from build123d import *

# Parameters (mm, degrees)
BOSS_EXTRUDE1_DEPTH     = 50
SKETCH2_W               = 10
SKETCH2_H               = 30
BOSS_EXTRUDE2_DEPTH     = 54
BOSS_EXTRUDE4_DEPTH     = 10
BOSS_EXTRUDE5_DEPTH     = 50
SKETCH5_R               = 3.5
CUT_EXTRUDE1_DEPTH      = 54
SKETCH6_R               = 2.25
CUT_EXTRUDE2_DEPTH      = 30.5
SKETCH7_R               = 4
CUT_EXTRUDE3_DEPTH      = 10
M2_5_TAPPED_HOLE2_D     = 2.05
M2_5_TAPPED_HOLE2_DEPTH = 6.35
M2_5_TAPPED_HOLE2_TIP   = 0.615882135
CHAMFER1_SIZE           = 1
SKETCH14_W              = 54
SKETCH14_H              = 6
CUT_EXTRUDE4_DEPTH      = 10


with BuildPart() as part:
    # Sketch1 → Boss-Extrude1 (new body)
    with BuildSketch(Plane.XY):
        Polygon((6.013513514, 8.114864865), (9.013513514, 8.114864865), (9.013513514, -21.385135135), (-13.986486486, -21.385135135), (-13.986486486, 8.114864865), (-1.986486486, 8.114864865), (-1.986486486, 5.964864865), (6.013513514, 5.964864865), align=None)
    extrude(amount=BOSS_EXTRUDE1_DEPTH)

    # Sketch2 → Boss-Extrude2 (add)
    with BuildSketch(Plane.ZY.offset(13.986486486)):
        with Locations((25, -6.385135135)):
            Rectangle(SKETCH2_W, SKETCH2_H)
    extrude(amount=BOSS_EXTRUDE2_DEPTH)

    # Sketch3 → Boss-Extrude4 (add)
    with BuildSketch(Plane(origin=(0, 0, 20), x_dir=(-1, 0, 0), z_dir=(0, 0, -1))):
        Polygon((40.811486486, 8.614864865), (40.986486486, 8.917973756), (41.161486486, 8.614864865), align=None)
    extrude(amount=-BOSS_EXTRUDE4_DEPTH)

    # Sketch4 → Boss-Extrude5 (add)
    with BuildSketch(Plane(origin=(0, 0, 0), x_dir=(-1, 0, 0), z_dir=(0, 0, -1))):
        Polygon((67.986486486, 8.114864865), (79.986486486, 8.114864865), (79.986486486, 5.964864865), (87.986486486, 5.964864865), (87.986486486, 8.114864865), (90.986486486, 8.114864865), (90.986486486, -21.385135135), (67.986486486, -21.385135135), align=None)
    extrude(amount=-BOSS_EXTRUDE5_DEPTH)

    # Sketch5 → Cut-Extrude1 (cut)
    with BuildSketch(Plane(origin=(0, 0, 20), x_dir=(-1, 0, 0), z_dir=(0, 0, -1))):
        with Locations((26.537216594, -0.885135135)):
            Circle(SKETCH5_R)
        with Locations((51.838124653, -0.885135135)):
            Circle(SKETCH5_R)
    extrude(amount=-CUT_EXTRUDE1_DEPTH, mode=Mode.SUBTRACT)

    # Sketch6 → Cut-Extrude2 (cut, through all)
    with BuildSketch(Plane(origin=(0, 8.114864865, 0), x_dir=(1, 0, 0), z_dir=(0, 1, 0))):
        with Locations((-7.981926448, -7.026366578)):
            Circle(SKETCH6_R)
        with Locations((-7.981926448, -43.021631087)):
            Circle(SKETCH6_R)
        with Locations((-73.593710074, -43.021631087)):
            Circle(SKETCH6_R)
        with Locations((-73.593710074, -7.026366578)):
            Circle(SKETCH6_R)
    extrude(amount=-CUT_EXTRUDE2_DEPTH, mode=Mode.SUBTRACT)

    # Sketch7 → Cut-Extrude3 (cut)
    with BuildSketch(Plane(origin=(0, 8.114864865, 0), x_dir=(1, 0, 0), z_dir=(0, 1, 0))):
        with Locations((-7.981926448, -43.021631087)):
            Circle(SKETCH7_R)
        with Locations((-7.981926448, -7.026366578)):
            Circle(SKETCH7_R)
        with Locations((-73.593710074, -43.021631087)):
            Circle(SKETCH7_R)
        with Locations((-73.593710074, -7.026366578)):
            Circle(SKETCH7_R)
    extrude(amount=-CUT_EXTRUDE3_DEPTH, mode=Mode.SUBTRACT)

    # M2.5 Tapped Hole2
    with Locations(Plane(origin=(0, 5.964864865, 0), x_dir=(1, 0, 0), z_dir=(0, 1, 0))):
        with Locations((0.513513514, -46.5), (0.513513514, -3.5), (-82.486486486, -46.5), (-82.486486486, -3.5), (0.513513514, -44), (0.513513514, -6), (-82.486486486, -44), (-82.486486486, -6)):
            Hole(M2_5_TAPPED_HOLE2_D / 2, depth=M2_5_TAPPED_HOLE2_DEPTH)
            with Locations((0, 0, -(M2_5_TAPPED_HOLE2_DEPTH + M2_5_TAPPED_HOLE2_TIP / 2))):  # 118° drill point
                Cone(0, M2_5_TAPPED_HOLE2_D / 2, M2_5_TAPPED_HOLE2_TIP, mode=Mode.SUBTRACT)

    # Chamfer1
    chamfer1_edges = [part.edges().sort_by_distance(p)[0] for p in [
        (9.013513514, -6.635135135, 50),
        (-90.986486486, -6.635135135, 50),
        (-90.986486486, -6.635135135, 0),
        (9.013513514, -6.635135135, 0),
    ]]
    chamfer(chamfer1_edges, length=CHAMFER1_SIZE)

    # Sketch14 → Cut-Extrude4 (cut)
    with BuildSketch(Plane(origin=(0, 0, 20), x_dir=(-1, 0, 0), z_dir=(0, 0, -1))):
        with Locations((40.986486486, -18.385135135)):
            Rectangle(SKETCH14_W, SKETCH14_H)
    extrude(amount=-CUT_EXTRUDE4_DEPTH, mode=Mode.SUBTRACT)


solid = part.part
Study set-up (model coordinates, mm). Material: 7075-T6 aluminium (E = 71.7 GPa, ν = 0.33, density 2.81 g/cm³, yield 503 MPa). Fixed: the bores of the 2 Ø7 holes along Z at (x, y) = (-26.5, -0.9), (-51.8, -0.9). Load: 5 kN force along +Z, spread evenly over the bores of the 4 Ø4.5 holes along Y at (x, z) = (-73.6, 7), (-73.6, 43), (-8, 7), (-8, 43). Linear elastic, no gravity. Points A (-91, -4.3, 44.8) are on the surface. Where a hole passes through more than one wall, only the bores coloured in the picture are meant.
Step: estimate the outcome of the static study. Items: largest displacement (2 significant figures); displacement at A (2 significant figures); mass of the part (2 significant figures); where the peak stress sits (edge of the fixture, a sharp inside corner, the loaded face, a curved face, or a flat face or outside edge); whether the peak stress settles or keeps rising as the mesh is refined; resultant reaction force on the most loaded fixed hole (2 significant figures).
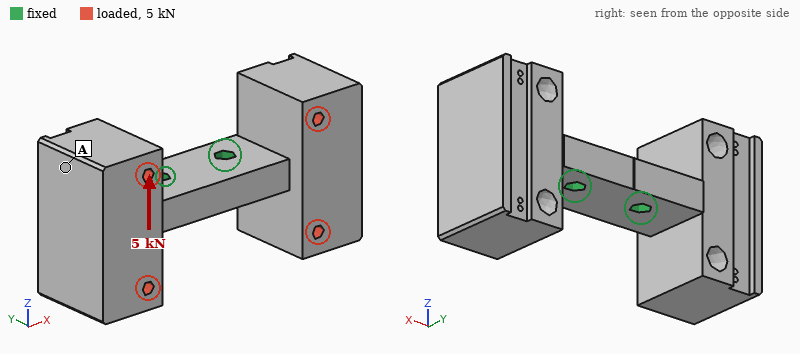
0.20 mm
0.16 mm
210 g
edge of the fixture
keeps rising
2.6 kN
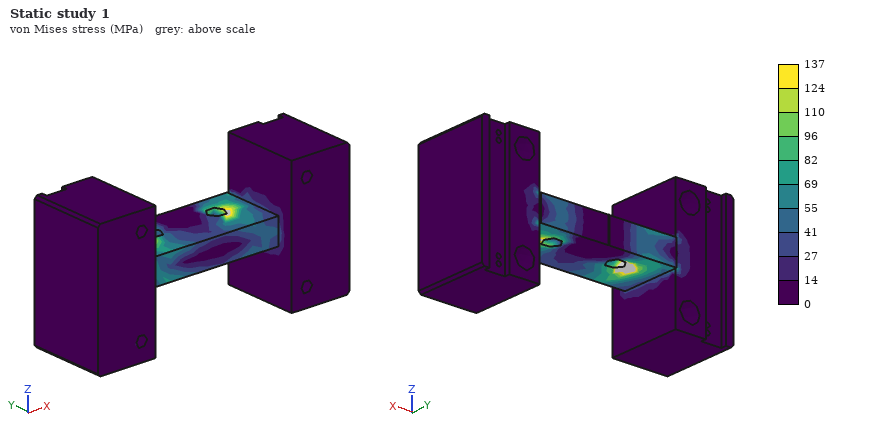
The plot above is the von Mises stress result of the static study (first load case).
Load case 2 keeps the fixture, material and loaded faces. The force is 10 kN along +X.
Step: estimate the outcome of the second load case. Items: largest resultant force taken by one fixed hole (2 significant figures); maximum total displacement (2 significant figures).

5.5 kN
68 µm
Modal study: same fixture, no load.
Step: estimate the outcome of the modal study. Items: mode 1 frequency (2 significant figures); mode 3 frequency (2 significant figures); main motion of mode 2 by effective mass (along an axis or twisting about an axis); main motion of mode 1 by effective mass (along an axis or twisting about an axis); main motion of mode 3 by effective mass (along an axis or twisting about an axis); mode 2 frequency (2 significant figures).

1900 Hz
3400 Hz
along Z
along Z
twisting about X
2200 Hz
